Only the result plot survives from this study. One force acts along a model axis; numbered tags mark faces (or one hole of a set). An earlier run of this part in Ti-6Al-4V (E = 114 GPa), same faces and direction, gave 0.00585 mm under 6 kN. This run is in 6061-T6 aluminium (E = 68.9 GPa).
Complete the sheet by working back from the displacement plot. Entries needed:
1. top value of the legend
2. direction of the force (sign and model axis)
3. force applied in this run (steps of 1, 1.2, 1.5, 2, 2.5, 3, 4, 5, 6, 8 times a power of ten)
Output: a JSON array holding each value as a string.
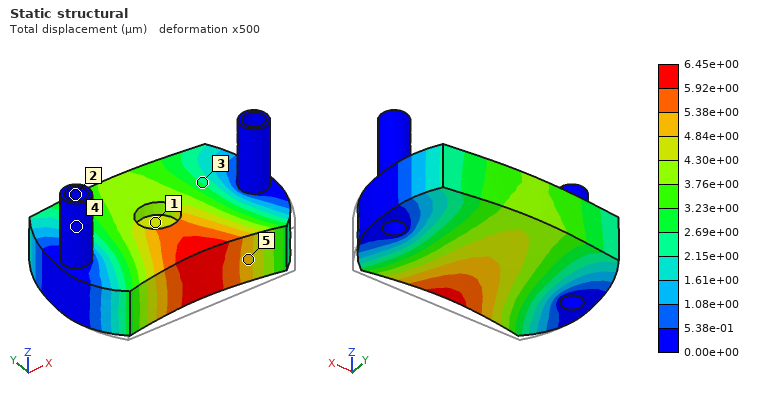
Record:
["6.45e+00 µm", "+Y", "4 kN"]
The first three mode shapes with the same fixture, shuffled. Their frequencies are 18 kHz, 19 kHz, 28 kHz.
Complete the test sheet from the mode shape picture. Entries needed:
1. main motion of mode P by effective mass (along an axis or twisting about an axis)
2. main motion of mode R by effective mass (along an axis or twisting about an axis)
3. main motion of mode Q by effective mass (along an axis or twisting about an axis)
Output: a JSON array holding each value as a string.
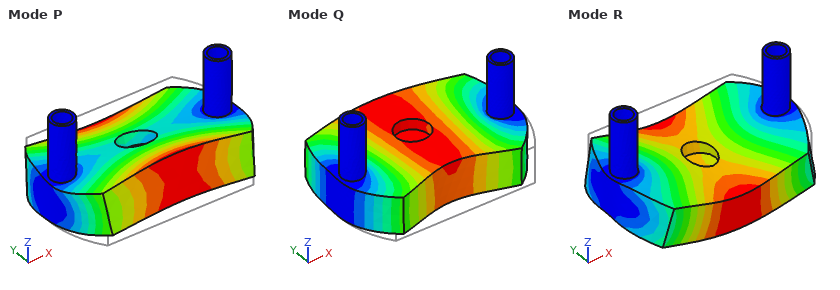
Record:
["twisting about X", "along Z", "along Y"]
